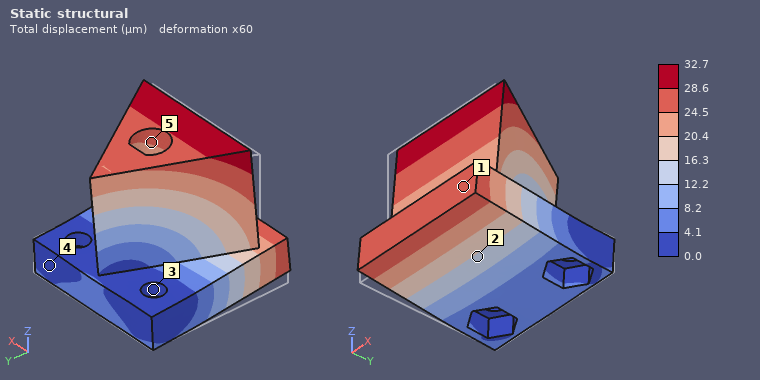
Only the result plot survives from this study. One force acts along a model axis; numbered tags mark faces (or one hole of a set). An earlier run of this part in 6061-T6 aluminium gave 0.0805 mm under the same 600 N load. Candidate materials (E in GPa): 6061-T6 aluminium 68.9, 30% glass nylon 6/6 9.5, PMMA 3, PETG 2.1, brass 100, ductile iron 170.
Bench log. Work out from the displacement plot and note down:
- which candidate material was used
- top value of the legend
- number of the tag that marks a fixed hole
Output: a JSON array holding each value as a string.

["ductile iron", "32.7 µm", "3"]
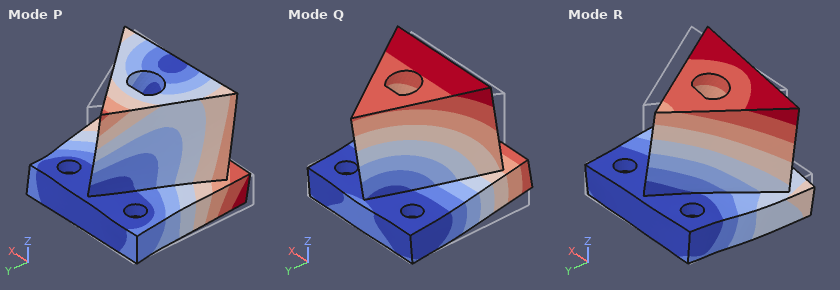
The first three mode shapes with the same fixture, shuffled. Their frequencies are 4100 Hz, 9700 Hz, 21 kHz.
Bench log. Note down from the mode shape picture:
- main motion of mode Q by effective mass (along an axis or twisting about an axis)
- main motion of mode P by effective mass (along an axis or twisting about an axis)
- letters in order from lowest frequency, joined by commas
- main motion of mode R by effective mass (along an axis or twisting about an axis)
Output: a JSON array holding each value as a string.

["along Z", "along X", "Q, R, P", "along X"]
